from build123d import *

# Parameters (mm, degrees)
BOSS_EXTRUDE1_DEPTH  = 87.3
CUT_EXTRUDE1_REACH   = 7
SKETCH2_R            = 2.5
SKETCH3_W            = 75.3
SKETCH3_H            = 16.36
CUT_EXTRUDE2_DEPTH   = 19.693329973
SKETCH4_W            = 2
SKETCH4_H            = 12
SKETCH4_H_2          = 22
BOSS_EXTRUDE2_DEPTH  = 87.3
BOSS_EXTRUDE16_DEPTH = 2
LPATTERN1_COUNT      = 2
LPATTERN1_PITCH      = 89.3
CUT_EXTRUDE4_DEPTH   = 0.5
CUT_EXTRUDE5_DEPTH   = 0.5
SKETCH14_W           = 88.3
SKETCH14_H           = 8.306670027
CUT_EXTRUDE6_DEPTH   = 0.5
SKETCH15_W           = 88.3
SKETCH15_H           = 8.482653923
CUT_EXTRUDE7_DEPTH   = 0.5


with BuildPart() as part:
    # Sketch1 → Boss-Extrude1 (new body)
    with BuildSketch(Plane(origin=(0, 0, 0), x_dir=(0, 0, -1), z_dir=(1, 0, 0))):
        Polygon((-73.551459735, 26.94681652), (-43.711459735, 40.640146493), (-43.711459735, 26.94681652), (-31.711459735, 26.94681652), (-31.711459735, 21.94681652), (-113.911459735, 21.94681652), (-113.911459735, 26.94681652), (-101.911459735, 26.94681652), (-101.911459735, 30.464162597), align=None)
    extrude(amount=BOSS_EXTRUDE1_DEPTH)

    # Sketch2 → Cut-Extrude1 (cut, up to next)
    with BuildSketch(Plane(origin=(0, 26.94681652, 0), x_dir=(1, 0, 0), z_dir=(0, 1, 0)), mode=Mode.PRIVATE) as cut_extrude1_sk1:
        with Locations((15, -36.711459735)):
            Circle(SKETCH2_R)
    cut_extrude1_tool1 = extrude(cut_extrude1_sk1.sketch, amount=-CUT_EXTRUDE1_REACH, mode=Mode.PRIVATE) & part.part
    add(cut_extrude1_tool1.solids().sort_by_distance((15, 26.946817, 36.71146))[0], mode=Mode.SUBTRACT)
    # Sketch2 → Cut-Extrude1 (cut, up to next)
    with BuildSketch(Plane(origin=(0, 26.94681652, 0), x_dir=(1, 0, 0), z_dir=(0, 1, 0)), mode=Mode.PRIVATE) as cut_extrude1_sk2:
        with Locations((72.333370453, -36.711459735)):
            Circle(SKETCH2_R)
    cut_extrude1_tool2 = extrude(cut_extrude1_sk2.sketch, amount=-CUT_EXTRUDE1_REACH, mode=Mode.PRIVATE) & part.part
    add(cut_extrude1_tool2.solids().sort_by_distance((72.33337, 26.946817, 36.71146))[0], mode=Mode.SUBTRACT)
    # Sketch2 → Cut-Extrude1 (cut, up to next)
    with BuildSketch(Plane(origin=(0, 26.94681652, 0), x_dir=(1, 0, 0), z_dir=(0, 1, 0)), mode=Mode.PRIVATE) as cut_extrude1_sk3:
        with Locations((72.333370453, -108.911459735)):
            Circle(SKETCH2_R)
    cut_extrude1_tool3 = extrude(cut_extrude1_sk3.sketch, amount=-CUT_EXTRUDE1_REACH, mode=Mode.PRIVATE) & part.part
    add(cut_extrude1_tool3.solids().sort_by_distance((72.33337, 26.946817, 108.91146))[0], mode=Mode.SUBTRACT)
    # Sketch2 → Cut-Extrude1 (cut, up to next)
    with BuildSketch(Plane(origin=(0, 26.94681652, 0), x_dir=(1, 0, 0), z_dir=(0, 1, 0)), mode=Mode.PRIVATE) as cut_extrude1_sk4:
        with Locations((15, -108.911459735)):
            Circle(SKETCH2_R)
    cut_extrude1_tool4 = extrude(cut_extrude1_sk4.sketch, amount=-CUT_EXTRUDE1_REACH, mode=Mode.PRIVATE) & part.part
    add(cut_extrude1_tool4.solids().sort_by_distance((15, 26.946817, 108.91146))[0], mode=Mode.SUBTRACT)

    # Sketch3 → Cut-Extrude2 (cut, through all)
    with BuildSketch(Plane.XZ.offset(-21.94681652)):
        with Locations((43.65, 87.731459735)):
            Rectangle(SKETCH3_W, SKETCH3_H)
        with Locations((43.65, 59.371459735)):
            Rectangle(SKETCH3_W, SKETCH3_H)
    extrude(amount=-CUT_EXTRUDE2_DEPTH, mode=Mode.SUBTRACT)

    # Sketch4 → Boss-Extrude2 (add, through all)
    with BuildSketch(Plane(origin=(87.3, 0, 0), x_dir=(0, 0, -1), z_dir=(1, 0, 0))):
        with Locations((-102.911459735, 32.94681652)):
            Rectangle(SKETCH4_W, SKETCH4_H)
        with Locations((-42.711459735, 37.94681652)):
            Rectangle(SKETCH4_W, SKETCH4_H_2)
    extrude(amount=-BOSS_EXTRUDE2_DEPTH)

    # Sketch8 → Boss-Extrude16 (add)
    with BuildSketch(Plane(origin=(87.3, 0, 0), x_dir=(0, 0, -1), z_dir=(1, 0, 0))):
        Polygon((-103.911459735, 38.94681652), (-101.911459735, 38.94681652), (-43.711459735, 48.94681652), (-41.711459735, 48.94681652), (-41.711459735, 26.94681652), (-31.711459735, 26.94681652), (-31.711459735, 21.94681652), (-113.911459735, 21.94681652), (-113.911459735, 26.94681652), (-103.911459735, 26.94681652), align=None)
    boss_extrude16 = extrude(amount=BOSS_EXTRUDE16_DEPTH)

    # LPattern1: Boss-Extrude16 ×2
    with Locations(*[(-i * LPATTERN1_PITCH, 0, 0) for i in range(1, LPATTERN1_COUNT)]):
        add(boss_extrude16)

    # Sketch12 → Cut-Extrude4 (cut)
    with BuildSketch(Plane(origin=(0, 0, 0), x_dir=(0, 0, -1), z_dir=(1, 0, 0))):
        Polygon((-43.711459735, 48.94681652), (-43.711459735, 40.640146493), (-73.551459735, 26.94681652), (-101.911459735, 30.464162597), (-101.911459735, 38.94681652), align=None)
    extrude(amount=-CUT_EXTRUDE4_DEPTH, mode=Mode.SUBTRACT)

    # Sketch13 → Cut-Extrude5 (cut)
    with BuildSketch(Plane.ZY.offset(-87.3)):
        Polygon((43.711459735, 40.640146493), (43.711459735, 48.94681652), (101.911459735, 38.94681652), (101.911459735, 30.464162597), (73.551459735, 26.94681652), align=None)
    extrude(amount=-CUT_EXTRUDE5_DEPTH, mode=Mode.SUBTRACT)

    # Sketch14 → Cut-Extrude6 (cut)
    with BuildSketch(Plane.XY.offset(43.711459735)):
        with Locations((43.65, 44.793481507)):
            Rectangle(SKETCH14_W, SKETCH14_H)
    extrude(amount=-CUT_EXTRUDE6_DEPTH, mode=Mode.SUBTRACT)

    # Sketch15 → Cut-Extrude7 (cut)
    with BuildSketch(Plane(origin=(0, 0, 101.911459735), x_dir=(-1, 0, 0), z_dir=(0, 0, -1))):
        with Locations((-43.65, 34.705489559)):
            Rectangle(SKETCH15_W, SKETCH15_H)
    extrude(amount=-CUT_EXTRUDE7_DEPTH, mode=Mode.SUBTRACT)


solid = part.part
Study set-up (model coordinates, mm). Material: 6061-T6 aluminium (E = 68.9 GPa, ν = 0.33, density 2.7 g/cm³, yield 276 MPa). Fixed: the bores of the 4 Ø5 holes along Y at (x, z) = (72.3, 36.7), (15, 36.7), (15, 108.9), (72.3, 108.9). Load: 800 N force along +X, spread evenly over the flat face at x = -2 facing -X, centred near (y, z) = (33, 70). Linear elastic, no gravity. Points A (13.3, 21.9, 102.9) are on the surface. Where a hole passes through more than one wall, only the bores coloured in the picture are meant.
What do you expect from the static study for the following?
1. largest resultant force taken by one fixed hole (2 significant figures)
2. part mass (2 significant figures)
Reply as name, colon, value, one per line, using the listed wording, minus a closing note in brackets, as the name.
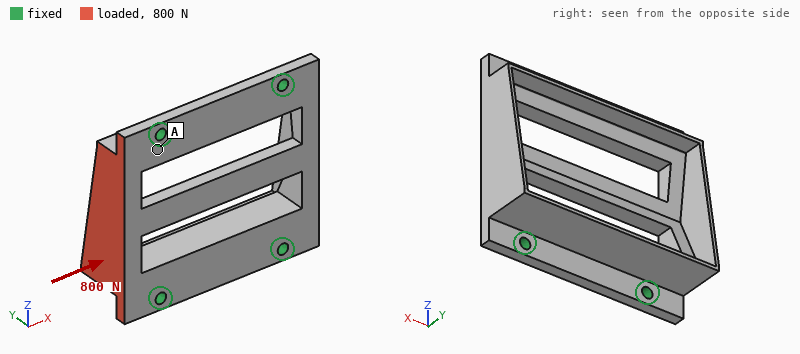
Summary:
largest resultant force taken by one fixed hole: 260 N
part mass: 120 g
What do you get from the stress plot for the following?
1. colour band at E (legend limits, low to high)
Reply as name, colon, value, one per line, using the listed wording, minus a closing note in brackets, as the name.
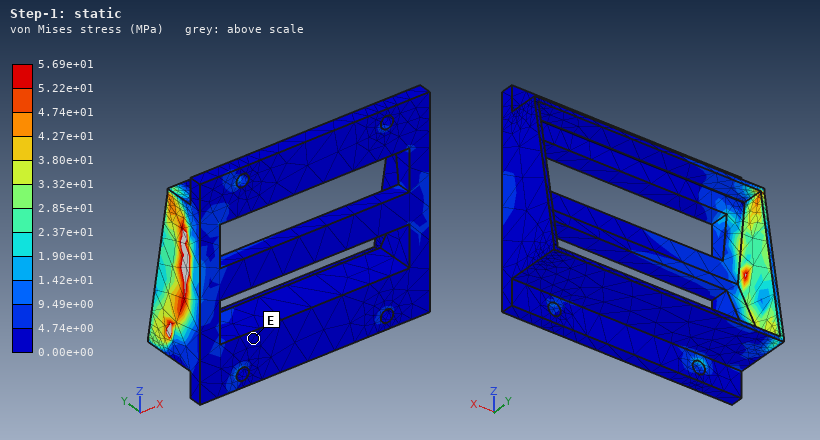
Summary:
colour band at E: 0.00e+00 to 4.74e+00 MPa
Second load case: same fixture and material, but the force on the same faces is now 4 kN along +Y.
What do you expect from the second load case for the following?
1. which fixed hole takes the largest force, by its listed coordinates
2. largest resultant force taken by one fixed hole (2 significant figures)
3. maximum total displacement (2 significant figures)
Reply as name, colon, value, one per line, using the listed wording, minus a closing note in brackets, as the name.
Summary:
which fixed hole takes the largest force, by its listed coordinates: (15, 36.7)
largest resultant force taken by one fixed hole: 3.1 kN
maximum total displacement: 0.24 mm
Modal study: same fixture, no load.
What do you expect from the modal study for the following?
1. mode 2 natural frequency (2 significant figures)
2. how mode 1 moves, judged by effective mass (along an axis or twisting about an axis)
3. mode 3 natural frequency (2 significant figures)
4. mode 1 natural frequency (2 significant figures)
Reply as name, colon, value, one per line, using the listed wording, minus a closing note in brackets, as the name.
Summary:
mode 2 natural frequency: 6000 Hz
how mode 1 moves, judged by effective mass: along Y
mode 3 natural frequency: 6100 Hz
mode 1 natural frequency: 3300 Hz
